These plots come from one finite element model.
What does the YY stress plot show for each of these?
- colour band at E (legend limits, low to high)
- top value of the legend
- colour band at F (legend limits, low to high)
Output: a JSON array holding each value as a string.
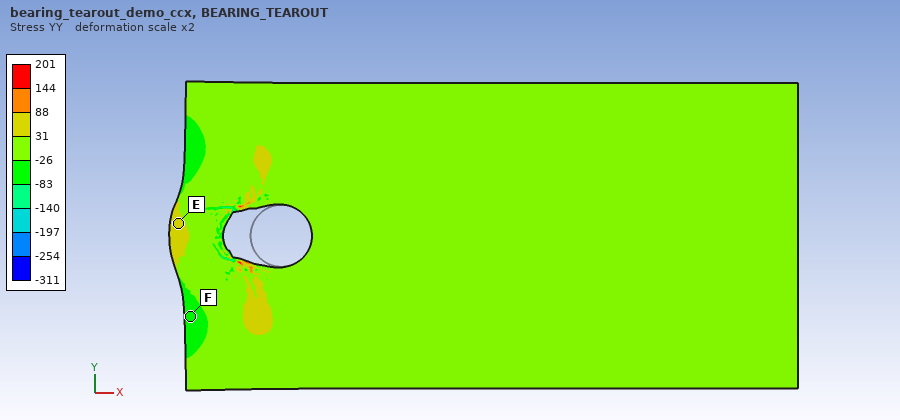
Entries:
["31 to 88", "201", "-83 to -26"]
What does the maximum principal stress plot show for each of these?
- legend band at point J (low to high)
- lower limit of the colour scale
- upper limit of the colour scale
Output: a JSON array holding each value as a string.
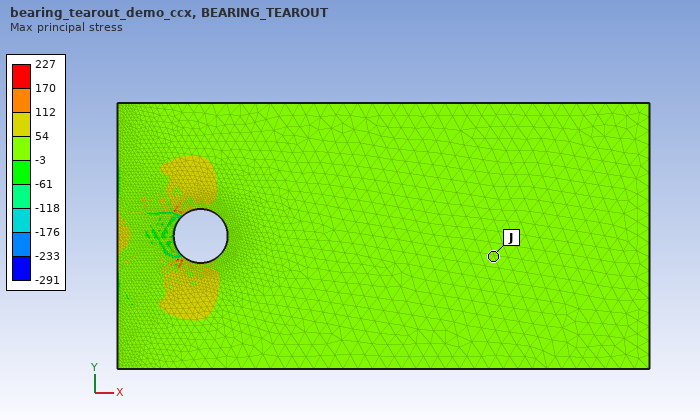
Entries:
["-3 to 54", "-291", "227"]
